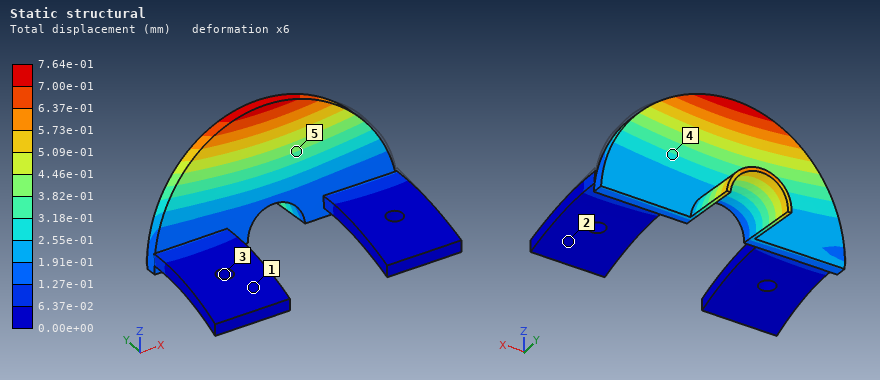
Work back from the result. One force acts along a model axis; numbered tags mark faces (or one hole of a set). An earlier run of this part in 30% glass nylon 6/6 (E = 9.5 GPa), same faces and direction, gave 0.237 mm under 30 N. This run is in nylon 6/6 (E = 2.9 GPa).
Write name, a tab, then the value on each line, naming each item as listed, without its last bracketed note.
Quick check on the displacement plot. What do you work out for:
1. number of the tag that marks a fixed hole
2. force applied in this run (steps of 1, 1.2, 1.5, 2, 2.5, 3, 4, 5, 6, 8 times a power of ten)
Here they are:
number of the tag that marks a fixed hole	3
force applied in this run	30 N
